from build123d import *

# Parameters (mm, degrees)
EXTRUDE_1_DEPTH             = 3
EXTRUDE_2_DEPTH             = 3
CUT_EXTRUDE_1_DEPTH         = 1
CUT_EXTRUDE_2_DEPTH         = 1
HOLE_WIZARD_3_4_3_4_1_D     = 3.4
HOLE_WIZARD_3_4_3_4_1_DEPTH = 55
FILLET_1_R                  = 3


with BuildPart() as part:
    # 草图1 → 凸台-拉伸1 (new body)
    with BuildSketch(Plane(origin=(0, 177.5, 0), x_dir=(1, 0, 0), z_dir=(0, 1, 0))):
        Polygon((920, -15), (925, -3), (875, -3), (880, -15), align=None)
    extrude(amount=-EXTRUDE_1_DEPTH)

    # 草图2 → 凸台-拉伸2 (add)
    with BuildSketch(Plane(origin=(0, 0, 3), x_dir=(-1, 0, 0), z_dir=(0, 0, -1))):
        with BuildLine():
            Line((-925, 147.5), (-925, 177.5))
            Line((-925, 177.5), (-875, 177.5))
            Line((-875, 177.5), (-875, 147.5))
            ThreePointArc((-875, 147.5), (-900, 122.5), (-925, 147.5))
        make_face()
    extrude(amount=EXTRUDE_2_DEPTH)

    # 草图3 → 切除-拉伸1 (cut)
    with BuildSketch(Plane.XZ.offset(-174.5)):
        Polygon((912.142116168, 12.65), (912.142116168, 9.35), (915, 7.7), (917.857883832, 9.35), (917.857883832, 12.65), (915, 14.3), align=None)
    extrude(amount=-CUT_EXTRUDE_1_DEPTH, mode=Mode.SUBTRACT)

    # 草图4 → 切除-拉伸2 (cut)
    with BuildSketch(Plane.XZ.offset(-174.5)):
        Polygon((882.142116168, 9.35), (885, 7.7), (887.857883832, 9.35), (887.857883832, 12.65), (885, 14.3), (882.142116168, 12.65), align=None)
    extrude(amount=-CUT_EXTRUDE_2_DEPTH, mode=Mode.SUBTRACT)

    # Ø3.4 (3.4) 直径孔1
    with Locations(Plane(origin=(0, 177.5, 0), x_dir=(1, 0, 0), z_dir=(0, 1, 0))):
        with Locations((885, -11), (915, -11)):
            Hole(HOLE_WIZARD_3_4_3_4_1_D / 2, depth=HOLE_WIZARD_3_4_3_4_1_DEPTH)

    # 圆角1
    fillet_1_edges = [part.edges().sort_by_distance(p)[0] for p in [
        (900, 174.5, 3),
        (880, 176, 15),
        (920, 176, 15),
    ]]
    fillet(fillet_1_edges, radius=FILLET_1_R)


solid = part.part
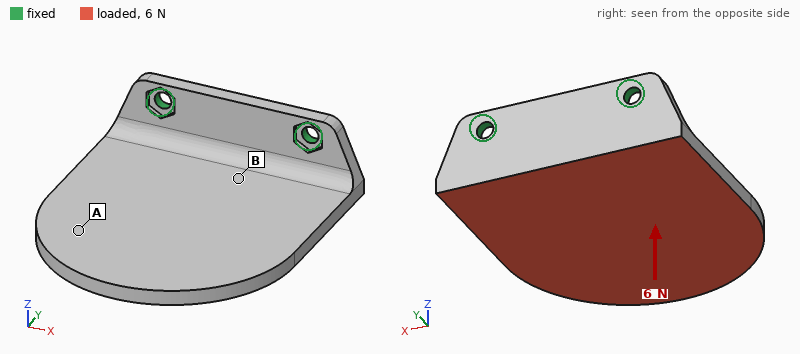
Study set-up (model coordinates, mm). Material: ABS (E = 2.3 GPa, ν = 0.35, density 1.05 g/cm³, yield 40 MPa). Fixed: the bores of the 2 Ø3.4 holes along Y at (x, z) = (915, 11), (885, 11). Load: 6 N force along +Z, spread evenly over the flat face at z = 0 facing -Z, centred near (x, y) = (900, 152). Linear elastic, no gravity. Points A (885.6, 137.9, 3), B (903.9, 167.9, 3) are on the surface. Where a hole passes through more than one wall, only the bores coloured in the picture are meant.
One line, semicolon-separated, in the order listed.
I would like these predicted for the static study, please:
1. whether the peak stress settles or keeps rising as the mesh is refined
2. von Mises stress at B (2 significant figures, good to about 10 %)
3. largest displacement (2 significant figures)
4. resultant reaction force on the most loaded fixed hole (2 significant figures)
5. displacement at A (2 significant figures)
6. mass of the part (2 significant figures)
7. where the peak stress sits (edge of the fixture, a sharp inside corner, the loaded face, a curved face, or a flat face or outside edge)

keeps rising; 1.3 MPa; 0.70 mm; 4.1 N; 0.47 mm; 9.5 g; edge of the fixture
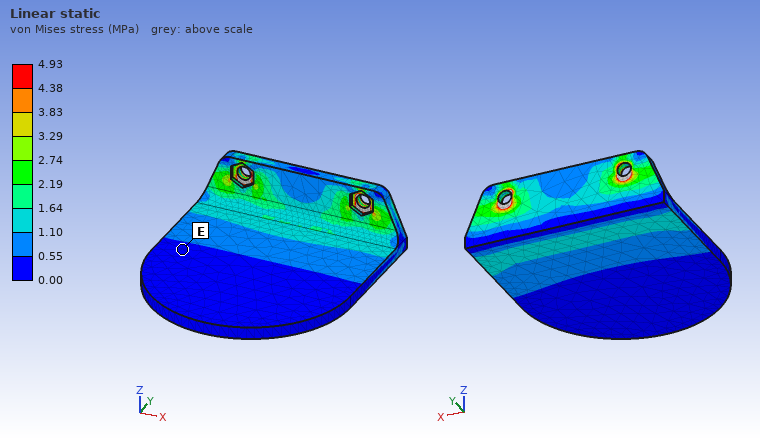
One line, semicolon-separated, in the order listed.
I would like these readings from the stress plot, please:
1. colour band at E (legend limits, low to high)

0.00 to 0.55 MPa
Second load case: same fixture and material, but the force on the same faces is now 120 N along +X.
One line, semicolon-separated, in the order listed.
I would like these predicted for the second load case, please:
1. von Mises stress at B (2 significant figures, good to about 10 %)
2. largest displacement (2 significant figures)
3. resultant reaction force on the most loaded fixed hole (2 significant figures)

5.0 MPa; 0.76 mm; 120 N
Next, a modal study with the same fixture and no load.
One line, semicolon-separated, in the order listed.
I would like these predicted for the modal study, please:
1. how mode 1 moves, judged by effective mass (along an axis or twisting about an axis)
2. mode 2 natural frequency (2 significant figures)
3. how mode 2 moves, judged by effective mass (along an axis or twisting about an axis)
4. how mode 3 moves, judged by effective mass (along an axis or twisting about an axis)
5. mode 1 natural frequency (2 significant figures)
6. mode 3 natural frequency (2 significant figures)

along Z; 650 Hz; along X; along X; 210 Hz; 1000 Hz
